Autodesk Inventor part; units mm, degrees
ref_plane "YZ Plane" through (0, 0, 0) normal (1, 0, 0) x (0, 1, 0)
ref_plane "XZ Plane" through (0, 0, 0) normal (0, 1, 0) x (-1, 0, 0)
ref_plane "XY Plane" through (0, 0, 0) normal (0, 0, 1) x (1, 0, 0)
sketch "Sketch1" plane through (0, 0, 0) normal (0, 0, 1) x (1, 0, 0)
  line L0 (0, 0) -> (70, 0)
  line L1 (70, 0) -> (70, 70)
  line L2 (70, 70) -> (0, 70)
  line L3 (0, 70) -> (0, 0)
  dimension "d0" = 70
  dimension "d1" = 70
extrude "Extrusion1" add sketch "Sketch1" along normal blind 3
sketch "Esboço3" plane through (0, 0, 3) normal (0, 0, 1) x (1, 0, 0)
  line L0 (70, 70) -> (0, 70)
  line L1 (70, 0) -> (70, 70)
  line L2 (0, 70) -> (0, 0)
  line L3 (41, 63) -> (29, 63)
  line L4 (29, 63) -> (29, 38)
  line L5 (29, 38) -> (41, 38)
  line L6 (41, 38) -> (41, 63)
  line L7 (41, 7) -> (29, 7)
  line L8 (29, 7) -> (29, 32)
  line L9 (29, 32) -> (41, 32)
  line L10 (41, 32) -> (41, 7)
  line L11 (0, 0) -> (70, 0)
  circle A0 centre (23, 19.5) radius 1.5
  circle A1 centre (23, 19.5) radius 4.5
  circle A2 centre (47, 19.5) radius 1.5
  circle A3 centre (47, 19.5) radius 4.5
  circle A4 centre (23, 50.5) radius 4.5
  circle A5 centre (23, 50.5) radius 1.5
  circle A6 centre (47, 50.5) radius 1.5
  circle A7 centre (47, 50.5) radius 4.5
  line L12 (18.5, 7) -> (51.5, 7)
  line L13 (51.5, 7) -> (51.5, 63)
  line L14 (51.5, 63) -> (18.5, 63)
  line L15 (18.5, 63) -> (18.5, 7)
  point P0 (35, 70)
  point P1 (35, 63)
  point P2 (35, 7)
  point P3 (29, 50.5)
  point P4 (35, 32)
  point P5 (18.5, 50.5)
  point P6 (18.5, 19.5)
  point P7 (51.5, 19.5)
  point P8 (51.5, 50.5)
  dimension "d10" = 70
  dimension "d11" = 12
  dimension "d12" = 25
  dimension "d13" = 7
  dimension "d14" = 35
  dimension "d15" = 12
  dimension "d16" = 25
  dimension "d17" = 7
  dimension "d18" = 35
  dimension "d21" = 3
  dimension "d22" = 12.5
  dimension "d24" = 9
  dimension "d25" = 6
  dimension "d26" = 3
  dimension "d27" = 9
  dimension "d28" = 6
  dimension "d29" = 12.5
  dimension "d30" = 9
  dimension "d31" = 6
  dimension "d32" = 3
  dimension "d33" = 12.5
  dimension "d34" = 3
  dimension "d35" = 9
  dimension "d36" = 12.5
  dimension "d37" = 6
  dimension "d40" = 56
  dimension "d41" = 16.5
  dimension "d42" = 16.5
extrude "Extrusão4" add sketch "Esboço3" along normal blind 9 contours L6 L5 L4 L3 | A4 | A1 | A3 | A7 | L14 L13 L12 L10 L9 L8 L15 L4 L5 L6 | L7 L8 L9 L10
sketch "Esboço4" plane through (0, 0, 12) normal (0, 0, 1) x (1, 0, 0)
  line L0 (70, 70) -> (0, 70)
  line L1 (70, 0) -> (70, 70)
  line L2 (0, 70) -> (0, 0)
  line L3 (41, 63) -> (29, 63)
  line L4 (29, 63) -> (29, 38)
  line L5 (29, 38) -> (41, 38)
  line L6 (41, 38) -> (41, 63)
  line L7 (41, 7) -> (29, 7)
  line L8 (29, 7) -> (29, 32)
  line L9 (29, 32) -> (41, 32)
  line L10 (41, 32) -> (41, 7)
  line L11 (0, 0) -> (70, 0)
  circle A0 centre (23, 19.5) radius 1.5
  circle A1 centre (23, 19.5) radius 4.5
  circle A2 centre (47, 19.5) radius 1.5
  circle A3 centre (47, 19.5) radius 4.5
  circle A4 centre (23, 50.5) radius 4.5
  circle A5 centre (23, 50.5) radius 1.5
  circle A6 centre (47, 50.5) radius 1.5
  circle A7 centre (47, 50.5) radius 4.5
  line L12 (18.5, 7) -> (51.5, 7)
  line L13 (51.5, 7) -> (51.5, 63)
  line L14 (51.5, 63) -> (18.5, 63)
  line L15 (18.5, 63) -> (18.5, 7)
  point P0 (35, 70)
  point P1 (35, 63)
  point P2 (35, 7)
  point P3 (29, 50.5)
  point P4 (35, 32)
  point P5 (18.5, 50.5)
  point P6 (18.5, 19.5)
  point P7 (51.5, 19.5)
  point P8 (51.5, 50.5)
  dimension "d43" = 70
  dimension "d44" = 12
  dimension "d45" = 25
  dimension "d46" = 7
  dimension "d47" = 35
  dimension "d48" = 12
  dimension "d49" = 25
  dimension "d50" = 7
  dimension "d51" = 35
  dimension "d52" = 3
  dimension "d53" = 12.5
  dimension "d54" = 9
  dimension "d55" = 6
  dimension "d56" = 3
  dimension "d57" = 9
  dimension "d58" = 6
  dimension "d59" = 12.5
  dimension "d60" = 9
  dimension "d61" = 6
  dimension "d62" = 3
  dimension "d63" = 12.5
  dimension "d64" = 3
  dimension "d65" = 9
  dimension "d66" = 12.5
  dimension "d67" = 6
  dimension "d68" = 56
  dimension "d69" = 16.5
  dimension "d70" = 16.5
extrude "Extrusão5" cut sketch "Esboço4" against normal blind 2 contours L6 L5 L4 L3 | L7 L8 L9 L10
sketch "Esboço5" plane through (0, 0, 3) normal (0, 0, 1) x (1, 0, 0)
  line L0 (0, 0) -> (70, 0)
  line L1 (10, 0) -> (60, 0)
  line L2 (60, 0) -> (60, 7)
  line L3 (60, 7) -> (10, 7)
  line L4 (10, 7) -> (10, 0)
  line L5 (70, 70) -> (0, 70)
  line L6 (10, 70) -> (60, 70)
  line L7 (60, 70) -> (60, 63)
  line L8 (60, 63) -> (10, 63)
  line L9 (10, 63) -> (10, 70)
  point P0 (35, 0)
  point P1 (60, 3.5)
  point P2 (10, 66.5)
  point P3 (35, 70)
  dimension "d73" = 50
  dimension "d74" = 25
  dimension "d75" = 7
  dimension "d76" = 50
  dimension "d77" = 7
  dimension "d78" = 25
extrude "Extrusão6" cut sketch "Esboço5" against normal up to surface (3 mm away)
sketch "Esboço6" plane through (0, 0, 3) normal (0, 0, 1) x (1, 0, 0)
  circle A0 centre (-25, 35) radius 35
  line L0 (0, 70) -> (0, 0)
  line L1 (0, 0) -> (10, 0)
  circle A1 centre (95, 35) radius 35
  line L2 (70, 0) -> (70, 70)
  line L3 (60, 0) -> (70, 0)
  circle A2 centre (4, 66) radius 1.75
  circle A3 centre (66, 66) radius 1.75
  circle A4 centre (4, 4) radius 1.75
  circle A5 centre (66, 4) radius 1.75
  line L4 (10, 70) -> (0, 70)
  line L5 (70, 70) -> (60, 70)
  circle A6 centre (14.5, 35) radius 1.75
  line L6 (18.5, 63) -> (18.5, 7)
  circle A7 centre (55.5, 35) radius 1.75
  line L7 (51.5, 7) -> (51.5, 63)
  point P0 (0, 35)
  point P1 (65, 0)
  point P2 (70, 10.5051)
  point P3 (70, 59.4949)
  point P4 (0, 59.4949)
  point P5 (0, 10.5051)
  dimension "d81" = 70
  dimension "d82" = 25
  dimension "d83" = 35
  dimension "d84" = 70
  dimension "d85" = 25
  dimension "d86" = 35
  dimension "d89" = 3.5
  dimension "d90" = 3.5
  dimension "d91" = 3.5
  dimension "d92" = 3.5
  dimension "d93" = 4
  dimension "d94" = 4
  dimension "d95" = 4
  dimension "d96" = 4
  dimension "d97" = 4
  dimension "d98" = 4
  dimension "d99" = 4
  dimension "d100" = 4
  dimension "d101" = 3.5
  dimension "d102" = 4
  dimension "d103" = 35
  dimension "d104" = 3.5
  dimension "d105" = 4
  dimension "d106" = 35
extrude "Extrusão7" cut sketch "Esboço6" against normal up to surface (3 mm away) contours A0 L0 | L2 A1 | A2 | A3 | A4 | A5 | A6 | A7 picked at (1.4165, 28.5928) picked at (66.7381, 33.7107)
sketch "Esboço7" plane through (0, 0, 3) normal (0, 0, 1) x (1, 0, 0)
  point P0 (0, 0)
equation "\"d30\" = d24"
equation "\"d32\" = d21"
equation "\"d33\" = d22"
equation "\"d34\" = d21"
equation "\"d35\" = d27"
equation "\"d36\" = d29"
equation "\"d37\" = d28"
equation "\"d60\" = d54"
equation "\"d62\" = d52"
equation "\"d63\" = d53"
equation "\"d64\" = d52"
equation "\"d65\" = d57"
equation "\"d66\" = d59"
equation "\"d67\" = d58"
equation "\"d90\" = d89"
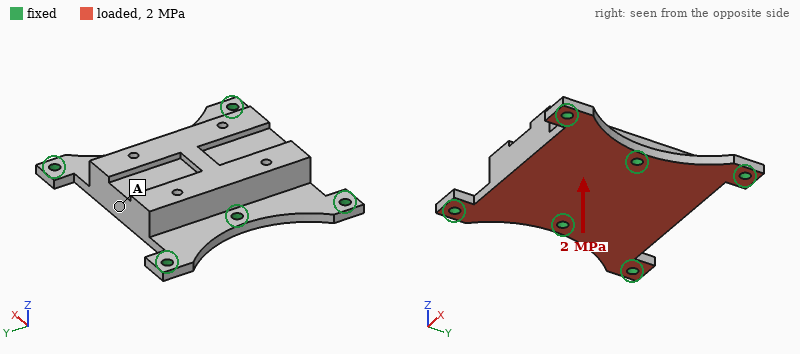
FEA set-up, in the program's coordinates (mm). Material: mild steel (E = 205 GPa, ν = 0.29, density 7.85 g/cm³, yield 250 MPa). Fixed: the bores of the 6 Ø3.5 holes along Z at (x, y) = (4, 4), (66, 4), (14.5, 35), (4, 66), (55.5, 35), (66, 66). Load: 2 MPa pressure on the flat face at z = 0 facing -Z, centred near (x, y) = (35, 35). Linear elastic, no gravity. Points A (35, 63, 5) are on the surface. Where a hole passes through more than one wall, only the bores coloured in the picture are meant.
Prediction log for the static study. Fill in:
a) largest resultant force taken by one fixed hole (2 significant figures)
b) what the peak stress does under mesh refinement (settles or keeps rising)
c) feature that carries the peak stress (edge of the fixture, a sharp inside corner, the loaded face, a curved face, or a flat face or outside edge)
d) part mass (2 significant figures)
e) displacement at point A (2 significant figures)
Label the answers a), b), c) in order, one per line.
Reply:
a) 2.9 kN
b) keeps rising
c) edge of the fixture
d) 200 g
e) 17 µm
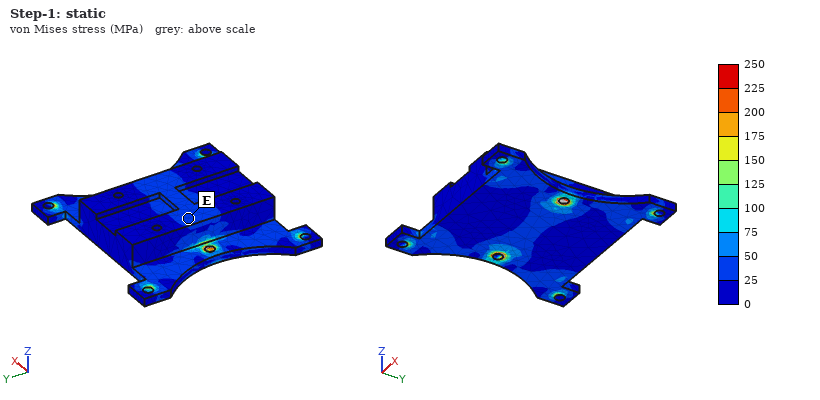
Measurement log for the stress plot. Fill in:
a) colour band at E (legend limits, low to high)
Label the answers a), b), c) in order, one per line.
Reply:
a) 25 to 50 MPa
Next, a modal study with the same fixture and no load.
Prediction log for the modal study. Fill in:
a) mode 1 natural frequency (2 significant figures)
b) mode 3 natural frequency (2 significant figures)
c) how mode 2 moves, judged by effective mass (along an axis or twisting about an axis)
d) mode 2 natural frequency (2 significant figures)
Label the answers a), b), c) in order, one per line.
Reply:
a) 4200 Hz
b) 13 kHz
c) along Z
d) 7500 Hz
